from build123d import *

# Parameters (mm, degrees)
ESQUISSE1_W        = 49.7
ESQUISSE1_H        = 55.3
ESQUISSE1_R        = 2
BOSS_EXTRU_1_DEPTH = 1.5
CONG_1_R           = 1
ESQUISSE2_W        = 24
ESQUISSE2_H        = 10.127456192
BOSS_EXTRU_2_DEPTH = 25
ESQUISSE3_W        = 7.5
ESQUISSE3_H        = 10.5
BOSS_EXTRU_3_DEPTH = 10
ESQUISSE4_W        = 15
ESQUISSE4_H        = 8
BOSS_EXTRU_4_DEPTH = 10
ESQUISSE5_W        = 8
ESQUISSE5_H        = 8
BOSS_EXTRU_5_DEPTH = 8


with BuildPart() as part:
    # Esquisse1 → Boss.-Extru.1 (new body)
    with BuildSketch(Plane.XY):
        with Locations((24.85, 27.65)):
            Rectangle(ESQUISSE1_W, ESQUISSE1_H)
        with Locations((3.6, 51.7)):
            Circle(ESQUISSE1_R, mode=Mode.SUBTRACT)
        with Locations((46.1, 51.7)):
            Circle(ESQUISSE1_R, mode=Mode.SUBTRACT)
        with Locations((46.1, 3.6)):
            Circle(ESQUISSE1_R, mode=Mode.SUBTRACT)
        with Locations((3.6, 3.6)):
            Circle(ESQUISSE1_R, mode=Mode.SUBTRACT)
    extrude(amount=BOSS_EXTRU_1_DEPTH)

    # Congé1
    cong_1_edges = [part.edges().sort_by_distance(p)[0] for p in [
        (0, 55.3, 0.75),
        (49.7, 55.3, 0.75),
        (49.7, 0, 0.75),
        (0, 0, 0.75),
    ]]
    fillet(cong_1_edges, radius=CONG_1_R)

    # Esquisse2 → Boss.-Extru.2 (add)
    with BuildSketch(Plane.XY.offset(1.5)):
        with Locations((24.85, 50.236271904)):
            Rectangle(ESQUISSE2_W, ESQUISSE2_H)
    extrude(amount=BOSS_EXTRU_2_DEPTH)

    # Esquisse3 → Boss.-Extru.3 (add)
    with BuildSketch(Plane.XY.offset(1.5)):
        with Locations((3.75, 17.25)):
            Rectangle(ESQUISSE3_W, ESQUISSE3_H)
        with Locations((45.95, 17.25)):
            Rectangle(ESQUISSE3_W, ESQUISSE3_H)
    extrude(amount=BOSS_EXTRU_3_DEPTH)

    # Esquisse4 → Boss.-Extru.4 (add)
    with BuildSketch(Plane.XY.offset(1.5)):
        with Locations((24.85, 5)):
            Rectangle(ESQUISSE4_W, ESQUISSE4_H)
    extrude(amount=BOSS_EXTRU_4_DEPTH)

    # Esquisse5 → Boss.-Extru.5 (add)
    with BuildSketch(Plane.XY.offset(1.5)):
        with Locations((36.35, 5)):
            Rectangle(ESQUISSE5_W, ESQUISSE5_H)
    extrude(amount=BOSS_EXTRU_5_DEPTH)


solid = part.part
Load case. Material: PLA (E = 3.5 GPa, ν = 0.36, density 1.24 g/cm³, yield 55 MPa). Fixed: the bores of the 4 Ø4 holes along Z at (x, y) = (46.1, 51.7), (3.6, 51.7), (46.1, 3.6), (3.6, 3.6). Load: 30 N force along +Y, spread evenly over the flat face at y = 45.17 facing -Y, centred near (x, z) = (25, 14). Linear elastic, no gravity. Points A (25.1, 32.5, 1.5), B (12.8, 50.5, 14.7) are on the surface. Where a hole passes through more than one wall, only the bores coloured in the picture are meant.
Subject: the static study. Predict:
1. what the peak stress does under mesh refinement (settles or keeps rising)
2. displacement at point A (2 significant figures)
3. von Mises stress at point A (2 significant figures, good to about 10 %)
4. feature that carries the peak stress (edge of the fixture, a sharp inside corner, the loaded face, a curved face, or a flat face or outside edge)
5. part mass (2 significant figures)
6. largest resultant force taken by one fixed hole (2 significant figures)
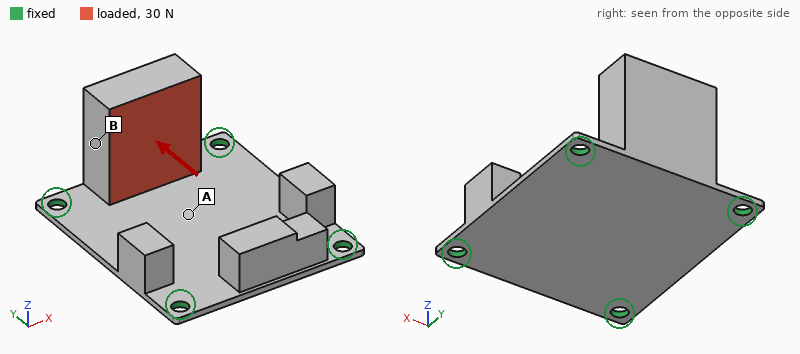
keeps rising
0.31 mm
5.0 MPa
edge of the fixture
17 g
12 N
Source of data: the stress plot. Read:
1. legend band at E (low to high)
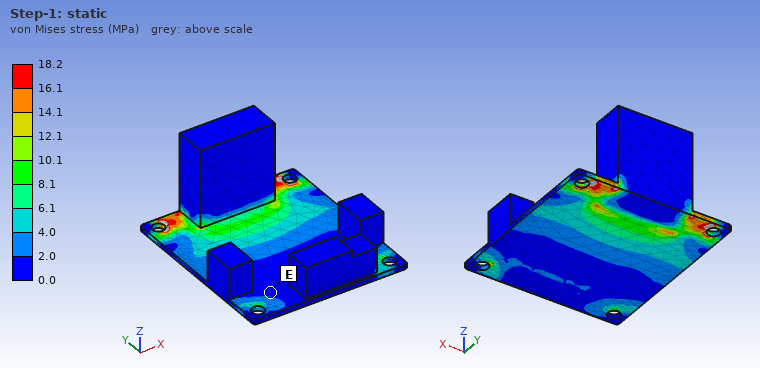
0.0 to 2.0 MPa
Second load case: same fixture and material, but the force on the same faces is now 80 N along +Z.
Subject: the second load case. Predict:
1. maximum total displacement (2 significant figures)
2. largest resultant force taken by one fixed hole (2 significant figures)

0.89 mm
40 N
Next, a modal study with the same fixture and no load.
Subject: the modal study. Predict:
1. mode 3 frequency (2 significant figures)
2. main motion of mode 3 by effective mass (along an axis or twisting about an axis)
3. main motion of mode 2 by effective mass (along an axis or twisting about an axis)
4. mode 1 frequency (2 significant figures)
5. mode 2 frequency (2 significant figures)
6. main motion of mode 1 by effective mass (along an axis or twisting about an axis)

1000 Hz
along X
along Z
380 Hz
930 Hz
along Y
